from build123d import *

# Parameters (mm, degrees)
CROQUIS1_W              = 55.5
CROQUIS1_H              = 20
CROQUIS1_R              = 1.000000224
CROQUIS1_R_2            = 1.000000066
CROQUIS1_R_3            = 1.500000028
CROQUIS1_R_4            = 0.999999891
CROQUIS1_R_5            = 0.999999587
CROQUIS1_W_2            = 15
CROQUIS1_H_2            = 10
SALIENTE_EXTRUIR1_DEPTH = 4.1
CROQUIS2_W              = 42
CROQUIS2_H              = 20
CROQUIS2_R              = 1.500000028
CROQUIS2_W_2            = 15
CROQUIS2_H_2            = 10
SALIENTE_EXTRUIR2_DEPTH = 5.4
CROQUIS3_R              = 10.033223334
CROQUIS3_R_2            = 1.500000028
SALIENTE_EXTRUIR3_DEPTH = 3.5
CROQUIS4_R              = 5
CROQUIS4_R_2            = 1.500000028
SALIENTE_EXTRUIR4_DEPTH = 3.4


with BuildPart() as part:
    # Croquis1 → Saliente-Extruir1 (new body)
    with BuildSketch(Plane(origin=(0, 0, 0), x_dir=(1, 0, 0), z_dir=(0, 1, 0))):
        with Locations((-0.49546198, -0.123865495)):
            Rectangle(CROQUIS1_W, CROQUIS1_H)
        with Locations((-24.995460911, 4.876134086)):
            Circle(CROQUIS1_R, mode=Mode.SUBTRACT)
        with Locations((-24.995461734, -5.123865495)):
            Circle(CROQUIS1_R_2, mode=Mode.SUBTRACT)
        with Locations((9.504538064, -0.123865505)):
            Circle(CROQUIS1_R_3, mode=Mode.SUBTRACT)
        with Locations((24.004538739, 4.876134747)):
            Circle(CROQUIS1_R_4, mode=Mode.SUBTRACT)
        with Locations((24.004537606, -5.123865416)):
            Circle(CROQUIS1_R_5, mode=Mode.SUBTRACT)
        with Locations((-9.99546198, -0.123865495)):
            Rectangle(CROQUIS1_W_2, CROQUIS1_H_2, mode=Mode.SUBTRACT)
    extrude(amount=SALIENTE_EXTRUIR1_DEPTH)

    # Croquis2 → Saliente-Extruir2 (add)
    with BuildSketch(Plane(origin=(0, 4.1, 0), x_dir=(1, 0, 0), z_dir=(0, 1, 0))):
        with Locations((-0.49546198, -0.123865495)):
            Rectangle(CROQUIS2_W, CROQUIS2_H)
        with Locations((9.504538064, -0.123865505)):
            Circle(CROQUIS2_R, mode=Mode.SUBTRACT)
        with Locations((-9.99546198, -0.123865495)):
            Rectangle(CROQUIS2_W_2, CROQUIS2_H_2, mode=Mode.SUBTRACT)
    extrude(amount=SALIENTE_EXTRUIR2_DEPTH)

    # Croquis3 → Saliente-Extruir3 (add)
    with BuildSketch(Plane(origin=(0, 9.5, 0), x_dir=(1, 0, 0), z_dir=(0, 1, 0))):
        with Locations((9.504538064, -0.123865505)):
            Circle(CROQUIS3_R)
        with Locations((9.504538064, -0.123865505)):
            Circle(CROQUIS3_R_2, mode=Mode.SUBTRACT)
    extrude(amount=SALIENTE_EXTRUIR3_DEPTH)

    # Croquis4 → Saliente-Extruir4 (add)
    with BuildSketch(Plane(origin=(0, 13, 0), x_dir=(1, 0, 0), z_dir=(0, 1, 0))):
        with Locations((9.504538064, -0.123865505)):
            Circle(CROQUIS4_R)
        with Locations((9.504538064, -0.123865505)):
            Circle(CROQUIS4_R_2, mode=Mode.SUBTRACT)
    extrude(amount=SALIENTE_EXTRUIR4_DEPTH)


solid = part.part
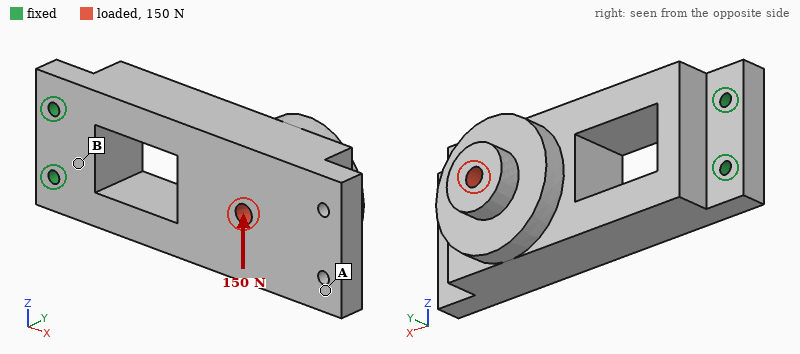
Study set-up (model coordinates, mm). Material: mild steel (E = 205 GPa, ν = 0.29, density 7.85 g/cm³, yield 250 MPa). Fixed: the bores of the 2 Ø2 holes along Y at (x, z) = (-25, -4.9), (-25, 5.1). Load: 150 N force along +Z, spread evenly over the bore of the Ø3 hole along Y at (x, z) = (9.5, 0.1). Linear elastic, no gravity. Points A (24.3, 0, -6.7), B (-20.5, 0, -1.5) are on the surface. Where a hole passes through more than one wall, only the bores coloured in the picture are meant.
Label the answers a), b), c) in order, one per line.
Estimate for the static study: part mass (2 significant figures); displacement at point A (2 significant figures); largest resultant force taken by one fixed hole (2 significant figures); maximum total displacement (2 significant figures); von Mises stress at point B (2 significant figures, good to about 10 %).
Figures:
a) 70 g
b) 10 µm
c) 460 N
d) 11 µm
e) 13 MPa
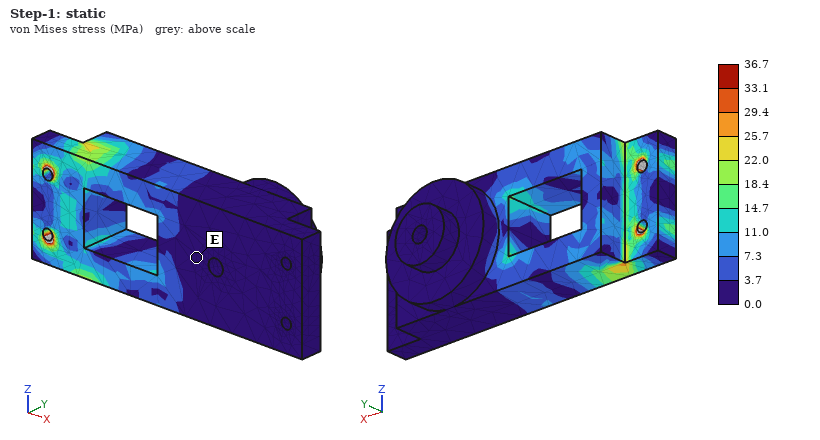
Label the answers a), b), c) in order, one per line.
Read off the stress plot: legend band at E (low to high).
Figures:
a) 0.0 to 3.7 MPa
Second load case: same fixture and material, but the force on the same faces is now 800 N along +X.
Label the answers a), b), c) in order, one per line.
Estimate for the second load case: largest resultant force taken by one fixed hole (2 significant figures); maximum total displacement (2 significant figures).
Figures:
a) 400 N
b) 81 µm
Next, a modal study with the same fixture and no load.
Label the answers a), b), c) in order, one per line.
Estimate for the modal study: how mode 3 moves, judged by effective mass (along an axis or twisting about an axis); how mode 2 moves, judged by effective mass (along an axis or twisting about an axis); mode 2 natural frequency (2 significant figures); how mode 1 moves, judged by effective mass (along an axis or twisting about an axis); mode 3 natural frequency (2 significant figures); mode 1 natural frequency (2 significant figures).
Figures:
a) twisting about X
b) along Z
c) 2900 Hz
d) along Y
e) 5900 Hz
f) 1100 Hz
